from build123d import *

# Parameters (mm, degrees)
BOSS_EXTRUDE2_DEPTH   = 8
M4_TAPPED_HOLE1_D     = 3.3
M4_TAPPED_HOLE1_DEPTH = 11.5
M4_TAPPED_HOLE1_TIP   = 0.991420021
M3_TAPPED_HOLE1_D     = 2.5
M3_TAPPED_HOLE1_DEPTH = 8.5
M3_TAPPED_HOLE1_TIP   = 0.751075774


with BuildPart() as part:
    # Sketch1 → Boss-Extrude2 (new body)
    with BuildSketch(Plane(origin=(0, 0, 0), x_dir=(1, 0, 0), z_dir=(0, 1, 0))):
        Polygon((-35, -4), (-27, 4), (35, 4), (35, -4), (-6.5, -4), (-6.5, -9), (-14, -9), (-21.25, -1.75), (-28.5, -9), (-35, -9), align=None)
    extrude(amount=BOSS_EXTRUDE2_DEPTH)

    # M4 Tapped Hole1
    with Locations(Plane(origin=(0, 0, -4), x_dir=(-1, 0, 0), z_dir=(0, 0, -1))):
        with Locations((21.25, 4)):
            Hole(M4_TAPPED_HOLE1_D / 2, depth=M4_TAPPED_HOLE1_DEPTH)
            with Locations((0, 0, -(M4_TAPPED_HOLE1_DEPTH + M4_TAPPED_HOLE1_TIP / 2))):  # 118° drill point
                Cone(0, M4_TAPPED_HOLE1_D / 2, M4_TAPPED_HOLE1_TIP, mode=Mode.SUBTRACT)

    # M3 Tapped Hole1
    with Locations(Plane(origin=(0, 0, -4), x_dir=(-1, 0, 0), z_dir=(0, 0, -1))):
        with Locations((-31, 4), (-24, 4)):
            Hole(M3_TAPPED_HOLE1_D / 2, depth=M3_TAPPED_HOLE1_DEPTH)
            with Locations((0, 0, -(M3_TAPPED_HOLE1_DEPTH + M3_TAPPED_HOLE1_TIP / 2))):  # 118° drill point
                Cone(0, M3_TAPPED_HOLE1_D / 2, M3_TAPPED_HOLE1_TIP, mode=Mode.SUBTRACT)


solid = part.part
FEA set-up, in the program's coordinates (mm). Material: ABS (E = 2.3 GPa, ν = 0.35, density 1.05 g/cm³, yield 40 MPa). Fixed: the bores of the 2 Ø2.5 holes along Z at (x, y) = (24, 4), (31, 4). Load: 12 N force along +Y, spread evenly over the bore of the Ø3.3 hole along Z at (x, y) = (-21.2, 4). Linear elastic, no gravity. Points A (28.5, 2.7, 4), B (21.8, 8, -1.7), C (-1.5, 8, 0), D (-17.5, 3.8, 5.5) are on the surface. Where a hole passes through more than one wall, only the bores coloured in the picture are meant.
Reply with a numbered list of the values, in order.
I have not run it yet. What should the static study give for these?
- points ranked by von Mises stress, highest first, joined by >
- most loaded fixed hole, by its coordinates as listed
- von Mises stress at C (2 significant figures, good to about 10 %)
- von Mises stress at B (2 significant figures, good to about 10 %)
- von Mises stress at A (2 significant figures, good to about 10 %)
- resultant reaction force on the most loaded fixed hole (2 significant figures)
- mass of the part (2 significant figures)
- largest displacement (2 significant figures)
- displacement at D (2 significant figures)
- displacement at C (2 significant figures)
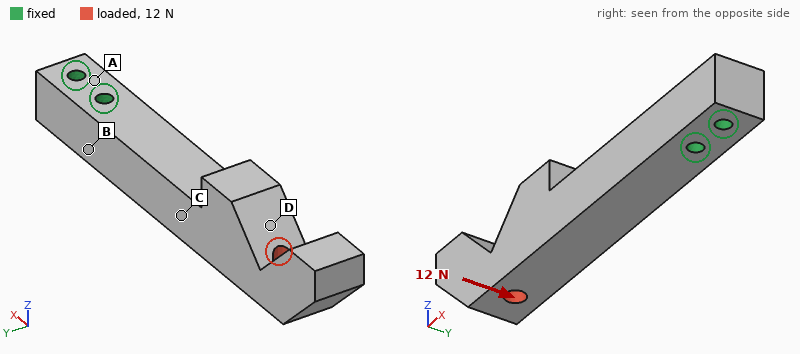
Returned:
1. B > C > A > D
2. (24, 4)
3. 2.8 MPa
4. 5.7 MPa
5. 1.7 MPa
6. 49 N
7. 5.1 g
8. 0.79 mm
9. 0.48 mm
10. 0.24 mm
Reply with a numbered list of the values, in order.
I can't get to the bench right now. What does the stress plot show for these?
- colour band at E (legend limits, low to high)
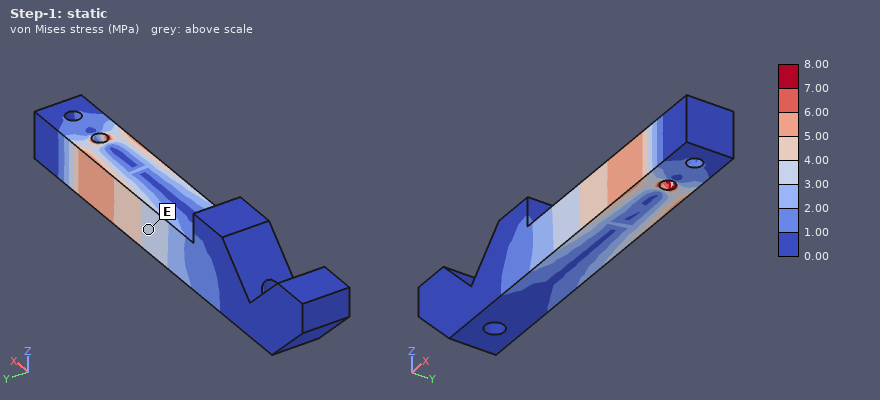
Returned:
1. 3.00 to 4.00 MPa
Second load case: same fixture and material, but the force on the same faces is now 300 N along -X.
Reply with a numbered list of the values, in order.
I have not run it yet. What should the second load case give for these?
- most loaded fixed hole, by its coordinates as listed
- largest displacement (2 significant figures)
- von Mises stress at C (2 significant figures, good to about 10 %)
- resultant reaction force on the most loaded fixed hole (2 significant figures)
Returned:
1. (24, 4)
2. 0.36 mm
3. 4.7 MPa
4. 260 N
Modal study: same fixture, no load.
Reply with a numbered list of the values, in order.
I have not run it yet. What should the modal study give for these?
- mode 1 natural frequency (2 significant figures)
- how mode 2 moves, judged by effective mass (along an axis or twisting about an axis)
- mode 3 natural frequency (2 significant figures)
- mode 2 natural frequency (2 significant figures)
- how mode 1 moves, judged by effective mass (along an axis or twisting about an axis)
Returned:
1. 480 Hz
2. along Z
3. 2600 Hz
4. 510 Hz
5. along Y
